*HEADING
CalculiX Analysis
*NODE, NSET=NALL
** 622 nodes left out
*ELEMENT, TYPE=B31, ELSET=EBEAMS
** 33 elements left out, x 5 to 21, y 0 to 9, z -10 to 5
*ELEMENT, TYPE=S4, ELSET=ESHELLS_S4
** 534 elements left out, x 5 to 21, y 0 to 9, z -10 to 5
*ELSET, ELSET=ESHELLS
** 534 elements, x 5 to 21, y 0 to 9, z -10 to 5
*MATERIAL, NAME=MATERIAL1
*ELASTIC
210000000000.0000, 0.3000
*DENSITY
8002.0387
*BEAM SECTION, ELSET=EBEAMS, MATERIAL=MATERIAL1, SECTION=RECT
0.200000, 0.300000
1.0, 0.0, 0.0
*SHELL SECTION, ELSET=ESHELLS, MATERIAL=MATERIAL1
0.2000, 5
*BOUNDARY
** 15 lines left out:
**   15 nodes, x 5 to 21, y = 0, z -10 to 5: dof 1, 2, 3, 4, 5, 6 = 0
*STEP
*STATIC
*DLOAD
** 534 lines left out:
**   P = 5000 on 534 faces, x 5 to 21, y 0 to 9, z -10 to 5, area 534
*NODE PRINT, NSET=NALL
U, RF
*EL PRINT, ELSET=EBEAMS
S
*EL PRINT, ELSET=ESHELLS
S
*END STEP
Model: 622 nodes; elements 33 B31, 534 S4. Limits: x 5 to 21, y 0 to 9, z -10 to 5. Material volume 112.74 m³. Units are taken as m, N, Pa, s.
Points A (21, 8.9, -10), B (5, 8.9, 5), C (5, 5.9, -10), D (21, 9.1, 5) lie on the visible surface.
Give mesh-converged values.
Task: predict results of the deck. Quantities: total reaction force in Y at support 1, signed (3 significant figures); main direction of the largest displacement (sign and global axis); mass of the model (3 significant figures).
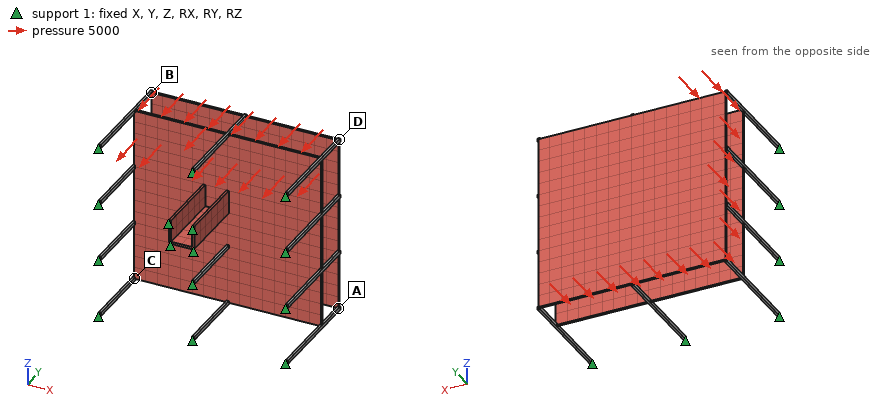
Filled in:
2.40e+06 N
-Y
9.02e+05 kg
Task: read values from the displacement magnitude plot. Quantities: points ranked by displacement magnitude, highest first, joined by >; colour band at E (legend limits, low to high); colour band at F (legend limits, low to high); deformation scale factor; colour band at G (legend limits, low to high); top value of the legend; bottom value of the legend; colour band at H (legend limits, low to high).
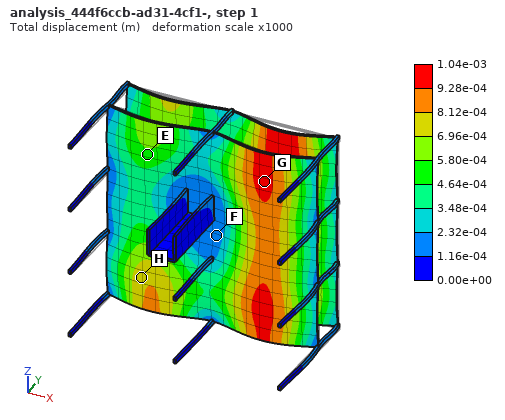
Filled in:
G > H > E > F
4.64e-04 to 5.80e-04 m
1.16e-04 to 2.32e-04 m
1000
9.28e-04 to 1.04e-03 m
1.04e-03 m
0.00e+00 m
6.96e-04 to 8.12e-04 m
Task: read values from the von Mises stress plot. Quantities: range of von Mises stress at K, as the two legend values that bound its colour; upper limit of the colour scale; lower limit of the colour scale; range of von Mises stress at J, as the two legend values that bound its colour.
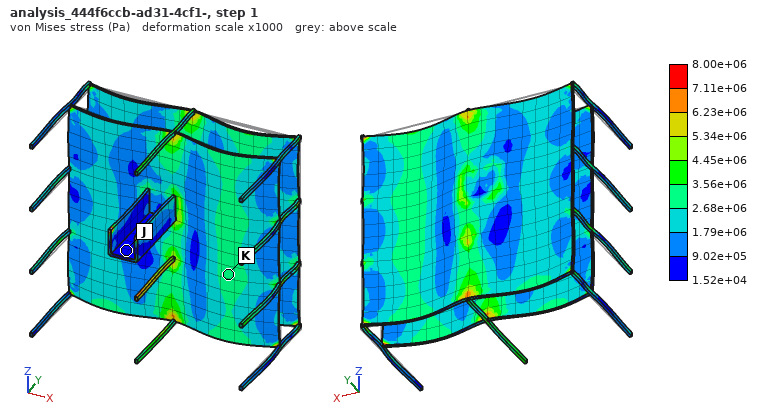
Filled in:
2.68e+06 to 3.56e+06 Pa
8.00e+06 Pa
1.52e+04 Pa
1.52e+04 to 9.02e+05 Pa
